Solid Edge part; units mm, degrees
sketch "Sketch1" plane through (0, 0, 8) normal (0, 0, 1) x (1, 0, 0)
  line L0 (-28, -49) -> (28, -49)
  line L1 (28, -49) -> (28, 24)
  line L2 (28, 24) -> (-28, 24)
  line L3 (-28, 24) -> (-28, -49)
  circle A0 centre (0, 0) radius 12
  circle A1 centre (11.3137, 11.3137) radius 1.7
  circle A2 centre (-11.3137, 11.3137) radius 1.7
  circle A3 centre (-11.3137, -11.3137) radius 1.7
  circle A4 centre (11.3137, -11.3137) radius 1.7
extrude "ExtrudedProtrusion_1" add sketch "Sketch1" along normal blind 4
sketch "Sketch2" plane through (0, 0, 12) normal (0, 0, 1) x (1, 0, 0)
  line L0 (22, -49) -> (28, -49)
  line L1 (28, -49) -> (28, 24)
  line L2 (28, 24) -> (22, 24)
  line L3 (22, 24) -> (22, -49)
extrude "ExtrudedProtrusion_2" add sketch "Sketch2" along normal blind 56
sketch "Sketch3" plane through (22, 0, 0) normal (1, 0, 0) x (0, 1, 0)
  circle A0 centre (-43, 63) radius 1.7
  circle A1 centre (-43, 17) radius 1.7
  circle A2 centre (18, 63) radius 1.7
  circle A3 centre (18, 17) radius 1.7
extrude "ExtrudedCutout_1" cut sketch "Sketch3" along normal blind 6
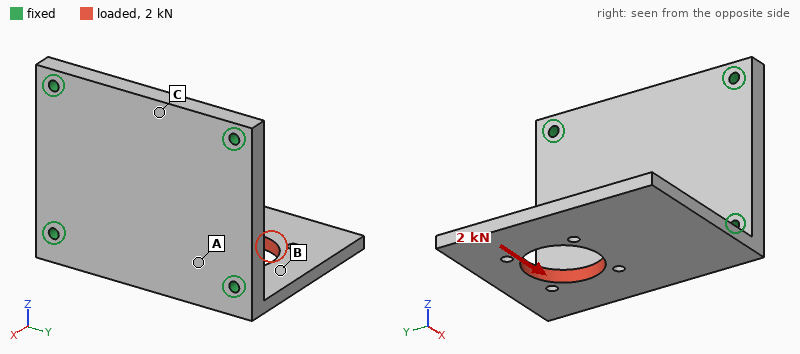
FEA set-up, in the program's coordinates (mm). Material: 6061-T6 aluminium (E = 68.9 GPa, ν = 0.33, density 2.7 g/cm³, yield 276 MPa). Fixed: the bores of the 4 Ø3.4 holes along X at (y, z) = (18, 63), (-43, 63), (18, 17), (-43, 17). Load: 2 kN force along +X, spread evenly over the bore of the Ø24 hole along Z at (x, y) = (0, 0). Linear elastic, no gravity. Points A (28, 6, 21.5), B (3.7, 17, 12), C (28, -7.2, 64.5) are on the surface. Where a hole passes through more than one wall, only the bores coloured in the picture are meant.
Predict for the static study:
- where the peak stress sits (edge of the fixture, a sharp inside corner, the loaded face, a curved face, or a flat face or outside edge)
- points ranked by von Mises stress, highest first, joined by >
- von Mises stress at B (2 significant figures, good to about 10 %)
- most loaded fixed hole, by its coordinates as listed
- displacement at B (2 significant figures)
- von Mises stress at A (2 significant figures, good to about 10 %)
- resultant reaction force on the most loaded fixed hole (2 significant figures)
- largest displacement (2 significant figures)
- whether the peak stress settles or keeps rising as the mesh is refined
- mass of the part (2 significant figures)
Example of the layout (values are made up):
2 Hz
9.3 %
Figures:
edge of the fixture
B > A > C
23 MPa
(18, 17)
36 µm
12 MPa
1.5 kN
78 µm
keeps rising
100 g
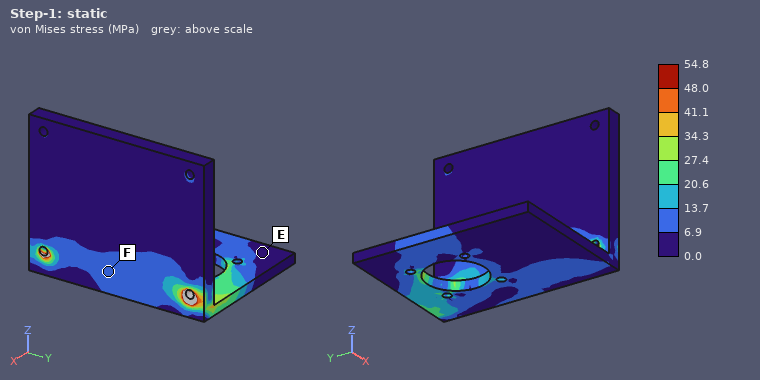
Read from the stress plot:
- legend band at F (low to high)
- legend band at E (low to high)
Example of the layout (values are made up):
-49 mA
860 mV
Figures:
6.9 to 13.7 MPa
0.0 to 6.9 MPa
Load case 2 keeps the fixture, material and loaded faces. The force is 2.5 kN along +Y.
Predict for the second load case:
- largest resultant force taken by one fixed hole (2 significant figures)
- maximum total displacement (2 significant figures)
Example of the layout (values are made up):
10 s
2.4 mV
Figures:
1.6 kN
55 µm
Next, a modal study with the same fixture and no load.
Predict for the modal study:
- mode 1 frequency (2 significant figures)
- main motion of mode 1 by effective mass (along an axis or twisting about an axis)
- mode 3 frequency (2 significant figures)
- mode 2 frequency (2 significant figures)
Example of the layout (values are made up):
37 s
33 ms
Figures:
1000 Hz
along Z
5000 Hz
2100 Hz
